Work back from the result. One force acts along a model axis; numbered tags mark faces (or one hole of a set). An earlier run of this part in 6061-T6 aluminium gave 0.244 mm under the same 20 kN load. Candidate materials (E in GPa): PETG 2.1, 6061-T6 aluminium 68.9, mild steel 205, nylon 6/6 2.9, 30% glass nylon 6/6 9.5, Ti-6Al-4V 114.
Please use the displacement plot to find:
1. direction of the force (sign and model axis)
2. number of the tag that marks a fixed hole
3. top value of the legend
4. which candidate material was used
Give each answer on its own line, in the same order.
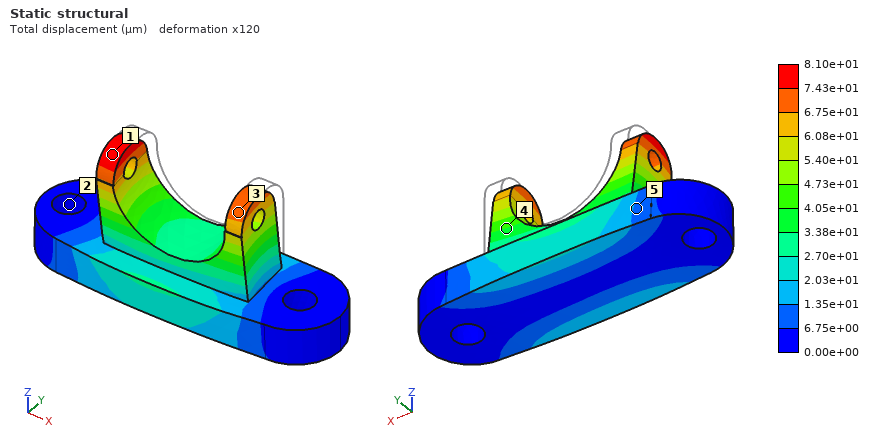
-Y
2
8.10e+01 µm
mild steel
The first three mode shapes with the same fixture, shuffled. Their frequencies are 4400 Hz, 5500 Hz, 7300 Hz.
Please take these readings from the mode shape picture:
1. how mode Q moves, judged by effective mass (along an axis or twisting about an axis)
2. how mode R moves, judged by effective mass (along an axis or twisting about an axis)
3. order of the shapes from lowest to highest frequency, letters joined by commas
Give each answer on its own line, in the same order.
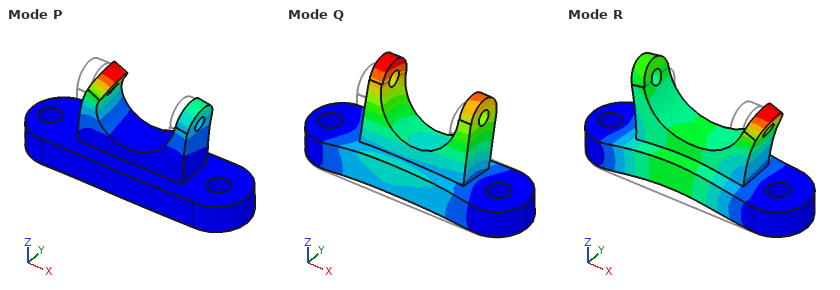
along Y
along Z
Q, R, P
